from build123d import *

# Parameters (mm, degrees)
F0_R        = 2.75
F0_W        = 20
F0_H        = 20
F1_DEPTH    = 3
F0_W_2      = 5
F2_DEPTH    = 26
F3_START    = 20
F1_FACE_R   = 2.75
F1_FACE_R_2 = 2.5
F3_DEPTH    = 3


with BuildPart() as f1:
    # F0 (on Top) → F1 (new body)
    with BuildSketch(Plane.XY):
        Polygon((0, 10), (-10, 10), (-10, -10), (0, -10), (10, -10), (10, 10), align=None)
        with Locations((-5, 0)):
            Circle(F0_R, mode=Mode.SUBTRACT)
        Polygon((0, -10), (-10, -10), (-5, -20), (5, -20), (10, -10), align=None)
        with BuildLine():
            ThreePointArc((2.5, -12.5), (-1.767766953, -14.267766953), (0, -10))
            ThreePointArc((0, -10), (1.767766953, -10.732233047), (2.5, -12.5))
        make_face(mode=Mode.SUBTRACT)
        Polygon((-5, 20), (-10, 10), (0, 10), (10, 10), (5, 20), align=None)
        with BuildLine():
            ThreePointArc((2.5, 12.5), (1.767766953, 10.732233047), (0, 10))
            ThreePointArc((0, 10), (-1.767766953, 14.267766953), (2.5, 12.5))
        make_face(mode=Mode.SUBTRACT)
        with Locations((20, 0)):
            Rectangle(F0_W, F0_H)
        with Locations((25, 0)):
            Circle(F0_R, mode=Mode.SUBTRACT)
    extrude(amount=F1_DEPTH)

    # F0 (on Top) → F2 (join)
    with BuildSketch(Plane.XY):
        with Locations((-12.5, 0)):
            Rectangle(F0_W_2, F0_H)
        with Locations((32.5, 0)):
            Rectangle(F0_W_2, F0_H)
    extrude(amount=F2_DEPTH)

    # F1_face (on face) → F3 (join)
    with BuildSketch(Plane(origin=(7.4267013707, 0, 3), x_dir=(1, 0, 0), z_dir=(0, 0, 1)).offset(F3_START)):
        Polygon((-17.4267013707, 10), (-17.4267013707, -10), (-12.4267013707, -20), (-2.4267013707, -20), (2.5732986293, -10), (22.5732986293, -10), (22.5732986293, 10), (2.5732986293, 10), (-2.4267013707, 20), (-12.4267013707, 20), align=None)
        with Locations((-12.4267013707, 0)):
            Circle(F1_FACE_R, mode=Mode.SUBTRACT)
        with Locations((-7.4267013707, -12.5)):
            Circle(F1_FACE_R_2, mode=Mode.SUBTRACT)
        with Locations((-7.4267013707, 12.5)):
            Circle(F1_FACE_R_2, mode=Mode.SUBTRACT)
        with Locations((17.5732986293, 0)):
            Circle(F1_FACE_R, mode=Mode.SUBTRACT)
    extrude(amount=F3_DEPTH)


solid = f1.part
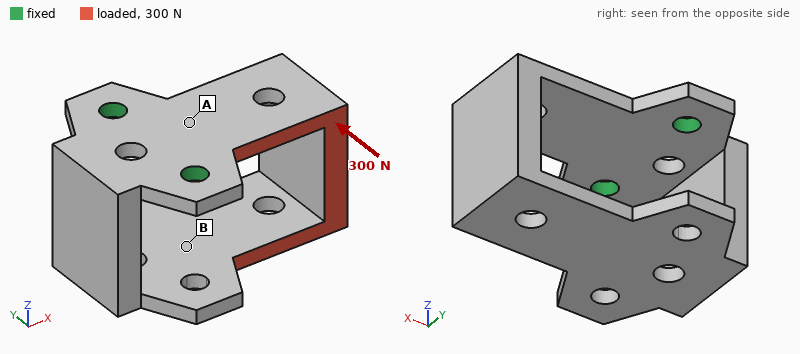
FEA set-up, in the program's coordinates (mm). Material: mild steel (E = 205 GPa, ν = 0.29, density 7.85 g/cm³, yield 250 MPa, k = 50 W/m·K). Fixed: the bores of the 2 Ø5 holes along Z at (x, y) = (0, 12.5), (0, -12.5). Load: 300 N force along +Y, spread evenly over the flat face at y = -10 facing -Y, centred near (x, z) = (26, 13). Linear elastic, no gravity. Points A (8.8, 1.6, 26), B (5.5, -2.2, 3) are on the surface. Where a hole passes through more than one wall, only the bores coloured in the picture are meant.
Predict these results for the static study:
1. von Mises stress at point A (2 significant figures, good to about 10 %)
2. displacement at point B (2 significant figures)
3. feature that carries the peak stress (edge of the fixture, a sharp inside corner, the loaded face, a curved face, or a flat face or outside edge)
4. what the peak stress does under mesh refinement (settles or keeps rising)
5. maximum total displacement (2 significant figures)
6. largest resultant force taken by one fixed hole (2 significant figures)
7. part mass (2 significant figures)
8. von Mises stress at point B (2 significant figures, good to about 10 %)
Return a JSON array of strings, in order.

["19 MPa", "23 µm", "a sharp inside corner", "keeps rising", "49 µm", "390 N", "89 g", "8.9 MPa"]
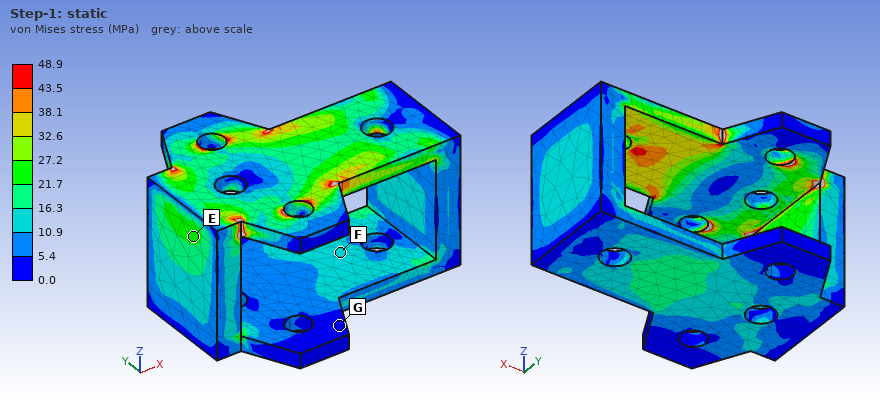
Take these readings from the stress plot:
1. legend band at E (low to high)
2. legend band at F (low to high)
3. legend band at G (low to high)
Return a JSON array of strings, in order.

["21.7 to 27.2 MPa", "10.9 to 16.3 MPa", "0.0 to 5.4 MPa"]
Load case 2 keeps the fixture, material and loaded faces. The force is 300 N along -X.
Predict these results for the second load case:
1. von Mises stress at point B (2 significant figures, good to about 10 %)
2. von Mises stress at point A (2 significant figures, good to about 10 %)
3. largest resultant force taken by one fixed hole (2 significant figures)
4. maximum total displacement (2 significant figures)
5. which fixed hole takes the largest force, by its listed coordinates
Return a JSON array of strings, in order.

["9.0 MPa", "29 MPa", "270 N", "73 µm", "(0, -12.5)"]
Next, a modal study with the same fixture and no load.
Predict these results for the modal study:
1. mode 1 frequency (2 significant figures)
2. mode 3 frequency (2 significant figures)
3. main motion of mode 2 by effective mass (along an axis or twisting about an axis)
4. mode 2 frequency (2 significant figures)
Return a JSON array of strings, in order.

["1000 Hz", "2600 Hz", "along Y", "2000 Hz"]
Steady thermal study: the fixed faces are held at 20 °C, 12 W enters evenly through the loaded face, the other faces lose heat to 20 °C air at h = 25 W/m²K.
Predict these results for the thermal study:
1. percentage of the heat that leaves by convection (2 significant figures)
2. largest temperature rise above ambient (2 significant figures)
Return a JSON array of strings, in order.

["41 %", "60 K"]
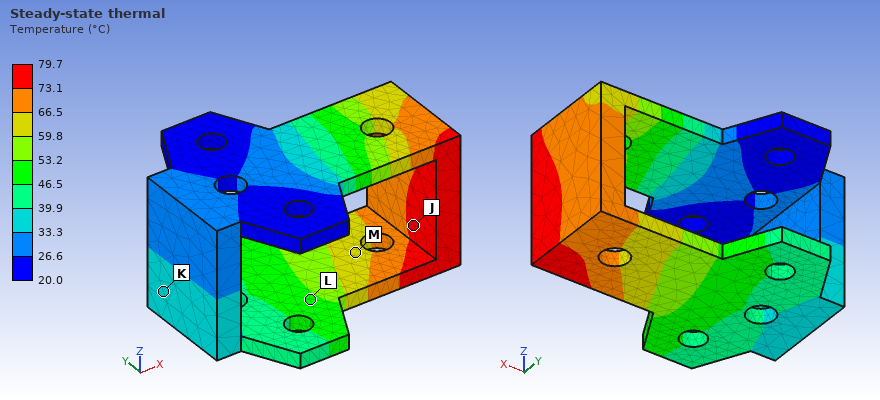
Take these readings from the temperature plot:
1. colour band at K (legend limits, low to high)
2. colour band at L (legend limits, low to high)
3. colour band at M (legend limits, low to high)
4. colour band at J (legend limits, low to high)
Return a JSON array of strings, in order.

["33.3 to 39.9 °C", "46.5 to 53.2 °C", "59.8 to 66.5 °C", "73.1 to 79.7 °C"]
